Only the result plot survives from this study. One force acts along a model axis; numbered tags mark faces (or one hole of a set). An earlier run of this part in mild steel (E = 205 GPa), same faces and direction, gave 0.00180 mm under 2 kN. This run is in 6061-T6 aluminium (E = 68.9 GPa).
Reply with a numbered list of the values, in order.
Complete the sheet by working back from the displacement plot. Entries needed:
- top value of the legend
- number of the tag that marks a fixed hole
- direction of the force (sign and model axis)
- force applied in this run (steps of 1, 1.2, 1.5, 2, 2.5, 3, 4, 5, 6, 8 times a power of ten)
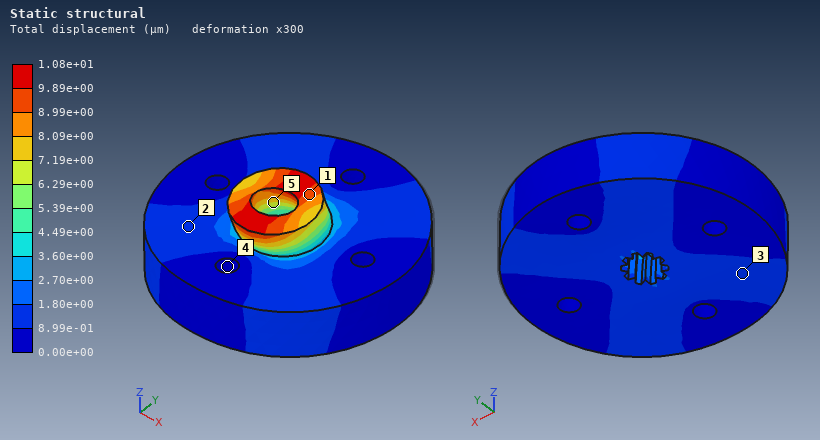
1. 1.08e+01 µm
2. 4
3. -Y
4. 4 kN
